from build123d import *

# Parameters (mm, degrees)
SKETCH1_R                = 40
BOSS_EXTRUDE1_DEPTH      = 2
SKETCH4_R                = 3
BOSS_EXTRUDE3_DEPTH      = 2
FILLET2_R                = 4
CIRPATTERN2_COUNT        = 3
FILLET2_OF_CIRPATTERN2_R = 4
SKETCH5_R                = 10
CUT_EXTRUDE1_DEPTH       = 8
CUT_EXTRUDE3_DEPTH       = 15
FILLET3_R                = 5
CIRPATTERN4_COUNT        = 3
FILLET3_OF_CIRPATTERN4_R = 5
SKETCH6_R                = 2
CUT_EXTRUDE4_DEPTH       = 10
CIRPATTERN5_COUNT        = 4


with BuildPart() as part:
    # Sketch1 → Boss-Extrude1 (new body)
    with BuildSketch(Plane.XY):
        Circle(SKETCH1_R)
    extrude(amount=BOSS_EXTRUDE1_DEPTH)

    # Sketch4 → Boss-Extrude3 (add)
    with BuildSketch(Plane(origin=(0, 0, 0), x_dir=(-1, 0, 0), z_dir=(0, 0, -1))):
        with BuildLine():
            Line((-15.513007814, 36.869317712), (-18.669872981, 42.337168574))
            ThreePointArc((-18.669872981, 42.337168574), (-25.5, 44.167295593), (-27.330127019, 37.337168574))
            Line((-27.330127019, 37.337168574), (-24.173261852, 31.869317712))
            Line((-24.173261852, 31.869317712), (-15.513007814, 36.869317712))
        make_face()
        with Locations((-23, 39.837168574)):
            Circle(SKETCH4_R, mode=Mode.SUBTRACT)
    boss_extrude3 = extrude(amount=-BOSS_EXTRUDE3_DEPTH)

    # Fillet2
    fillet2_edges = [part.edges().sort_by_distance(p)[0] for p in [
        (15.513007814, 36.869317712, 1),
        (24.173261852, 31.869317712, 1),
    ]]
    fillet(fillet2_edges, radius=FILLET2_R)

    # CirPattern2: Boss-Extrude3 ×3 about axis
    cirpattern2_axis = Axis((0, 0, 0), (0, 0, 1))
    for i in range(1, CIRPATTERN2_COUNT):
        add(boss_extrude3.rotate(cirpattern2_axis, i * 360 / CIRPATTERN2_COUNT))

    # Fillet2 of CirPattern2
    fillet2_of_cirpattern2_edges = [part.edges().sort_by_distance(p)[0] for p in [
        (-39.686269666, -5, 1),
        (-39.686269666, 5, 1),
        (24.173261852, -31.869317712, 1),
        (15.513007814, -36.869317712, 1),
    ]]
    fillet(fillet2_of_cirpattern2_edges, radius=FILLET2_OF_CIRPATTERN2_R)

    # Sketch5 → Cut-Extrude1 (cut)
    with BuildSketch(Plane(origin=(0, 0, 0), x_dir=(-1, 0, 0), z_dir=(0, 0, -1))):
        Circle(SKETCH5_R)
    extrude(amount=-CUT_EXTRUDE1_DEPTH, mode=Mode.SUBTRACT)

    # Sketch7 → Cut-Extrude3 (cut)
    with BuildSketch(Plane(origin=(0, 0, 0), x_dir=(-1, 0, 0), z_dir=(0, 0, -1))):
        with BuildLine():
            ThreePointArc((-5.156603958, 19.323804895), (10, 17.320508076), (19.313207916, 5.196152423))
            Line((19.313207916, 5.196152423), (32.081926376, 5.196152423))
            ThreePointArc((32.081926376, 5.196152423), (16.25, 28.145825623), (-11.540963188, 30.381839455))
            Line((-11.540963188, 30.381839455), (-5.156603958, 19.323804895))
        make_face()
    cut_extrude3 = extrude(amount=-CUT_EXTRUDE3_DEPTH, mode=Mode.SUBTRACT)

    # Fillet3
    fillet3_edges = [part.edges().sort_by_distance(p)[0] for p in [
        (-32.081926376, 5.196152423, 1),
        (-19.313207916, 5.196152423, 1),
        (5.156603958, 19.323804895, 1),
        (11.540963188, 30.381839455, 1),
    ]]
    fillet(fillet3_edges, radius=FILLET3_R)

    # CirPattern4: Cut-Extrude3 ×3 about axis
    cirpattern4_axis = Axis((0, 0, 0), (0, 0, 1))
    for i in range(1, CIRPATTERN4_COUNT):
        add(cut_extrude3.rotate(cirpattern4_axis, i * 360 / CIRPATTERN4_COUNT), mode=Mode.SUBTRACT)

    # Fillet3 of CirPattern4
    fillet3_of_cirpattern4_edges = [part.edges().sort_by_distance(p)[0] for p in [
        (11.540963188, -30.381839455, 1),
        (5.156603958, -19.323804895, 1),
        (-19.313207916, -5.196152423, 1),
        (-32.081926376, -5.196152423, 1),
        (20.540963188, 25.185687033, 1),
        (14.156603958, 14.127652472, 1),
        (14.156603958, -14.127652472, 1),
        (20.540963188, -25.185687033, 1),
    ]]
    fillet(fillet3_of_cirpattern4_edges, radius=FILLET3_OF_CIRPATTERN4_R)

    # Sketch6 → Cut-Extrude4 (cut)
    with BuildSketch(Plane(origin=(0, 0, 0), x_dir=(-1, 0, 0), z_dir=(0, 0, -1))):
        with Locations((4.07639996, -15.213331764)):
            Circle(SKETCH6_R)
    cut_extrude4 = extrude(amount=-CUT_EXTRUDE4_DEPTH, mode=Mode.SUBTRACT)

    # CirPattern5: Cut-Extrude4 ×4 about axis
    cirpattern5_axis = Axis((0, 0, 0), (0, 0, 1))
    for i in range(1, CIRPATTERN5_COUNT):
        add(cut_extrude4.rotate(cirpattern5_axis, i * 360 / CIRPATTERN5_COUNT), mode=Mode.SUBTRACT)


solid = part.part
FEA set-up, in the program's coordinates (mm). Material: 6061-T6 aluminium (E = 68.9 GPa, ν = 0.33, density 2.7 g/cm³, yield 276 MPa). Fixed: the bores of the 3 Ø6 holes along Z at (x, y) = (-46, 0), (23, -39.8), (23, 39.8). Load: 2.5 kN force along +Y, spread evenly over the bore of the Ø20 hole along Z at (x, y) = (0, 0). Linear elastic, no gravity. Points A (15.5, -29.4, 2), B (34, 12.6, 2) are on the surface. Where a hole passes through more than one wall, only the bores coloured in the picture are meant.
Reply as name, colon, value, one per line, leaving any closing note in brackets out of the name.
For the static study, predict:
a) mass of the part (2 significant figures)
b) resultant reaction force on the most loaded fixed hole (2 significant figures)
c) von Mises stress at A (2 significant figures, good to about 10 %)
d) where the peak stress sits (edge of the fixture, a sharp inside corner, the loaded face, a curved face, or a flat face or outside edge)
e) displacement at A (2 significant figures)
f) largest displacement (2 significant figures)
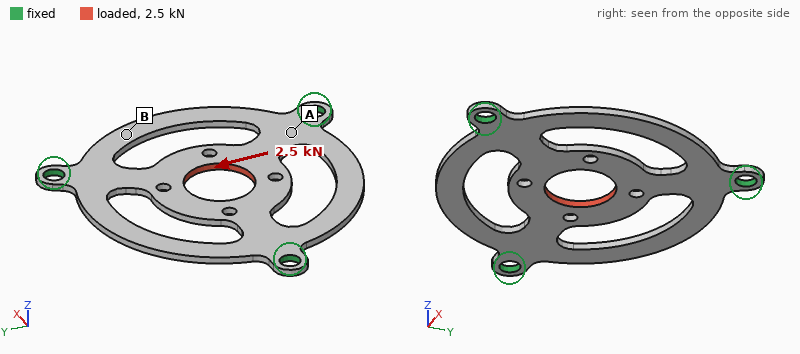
mass of the part: 18 g
resultant reaction force on the most loaded fixed hole: 1.1 kN
von Mises stress at A: 56 MPa
where the peak stress sits: a curved face
displacement at A: 13 µm
largest displacement: 76 µm
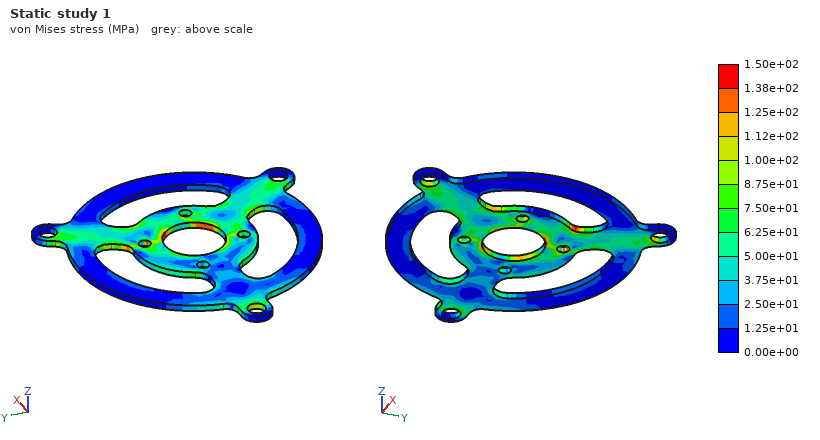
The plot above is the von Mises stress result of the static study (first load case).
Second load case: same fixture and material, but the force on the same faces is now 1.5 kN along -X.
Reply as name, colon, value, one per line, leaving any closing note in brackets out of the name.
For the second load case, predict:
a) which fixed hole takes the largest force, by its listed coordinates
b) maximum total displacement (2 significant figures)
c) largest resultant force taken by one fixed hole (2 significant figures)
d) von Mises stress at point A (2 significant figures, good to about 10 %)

which fixed hole takes the largest force, by its listed coordinates: (-46, 0)
maximum total displacement: 47 µm
largest resultant force taken by one fixed hole: 780 N
von Mises stress at point A: 16 MPa
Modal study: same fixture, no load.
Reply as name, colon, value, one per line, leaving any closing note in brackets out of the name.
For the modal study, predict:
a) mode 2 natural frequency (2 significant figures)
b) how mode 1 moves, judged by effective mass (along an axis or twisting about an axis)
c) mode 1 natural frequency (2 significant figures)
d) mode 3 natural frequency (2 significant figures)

mode 2 natural frequency: 1600 Hz
how mode 1 moves, judged by effective mass: along Z
mode 1 natural frequency: 1500 Hz
mode 3 natural frequency: 1600 Hz
